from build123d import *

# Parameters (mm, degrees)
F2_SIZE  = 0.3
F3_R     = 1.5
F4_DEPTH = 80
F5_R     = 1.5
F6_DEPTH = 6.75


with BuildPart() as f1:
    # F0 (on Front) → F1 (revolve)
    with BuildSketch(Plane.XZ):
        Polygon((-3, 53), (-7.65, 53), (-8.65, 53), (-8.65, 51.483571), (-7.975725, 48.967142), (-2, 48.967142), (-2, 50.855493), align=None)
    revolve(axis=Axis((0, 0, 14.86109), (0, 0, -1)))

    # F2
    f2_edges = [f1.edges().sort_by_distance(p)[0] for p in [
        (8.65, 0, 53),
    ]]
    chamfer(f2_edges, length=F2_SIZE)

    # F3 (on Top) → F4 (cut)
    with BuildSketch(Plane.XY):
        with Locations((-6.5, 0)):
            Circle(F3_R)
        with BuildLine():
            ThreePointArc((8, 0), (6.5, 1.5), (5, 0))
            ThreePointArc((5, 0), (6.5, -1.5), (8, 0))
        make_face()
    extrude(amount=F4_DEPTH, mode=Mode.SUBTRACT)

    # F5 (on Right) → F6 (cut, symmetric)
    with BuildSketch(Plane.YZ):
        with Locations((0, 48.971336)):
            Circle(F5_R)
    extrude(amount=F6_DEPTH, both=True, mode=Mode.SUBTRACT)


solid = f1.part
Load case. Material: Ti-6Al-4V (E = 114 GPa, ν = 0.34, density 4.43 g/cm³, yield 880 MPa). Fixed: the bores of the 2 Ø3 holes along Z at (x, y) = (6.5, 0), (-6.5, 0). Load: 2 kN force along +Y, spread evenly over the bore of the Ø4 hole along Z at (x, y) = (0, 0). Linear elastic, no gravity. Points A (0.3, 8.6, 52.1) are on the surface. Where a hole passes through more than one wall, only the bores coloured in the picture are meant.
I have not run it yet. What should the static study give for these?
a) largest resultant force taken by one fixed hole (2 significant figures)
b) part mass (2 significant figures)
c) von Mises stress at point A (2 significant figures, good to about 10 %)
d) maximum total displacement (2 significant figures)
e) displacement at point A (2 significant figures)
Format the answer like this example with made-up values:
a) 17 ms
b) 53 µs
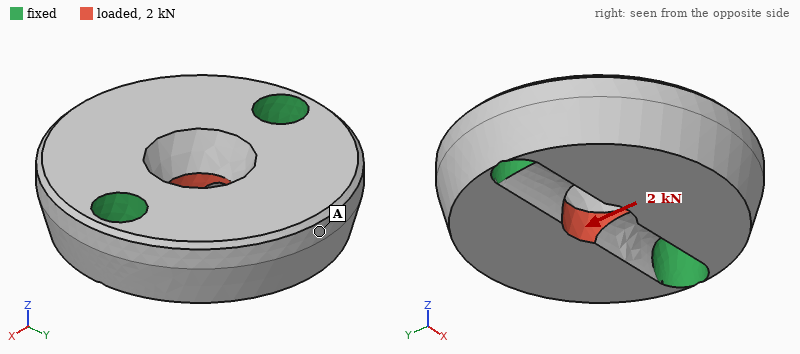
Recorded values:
a) 1.0 kN
b) 3.3 g
c) 31 MPa
d) 7.3 µm
e) 6.1 µm
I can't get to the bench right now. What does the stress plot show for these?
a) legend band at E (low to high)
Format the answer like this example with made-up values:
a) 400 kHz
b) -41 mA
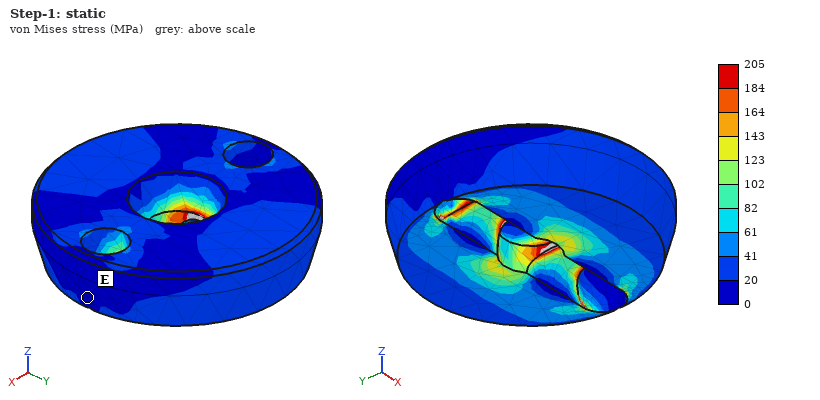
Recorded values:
a) 0 to 20 MPa
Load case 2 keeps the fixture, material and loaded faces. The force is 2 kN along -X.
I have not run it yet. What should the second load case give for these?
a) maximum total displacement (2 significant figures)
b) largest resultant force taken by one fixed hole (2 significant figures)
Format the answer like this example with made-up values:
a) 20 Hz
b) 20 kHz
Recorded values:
a) 4.3 µm
b) 1.0 kN
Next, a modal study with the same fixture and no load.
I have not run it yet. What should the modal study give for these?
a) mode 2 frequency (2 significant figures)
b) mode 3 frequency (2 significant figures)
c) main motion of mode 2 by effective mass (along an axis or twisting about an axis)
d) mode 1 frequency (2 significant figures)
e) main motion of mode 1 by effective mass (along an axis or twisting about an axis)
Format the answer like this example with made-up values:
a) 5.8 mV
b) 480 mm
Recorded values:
a) 42 kHz
b) 94 kHz
c) along Z
d) 40 kHz
e) twisting about X
